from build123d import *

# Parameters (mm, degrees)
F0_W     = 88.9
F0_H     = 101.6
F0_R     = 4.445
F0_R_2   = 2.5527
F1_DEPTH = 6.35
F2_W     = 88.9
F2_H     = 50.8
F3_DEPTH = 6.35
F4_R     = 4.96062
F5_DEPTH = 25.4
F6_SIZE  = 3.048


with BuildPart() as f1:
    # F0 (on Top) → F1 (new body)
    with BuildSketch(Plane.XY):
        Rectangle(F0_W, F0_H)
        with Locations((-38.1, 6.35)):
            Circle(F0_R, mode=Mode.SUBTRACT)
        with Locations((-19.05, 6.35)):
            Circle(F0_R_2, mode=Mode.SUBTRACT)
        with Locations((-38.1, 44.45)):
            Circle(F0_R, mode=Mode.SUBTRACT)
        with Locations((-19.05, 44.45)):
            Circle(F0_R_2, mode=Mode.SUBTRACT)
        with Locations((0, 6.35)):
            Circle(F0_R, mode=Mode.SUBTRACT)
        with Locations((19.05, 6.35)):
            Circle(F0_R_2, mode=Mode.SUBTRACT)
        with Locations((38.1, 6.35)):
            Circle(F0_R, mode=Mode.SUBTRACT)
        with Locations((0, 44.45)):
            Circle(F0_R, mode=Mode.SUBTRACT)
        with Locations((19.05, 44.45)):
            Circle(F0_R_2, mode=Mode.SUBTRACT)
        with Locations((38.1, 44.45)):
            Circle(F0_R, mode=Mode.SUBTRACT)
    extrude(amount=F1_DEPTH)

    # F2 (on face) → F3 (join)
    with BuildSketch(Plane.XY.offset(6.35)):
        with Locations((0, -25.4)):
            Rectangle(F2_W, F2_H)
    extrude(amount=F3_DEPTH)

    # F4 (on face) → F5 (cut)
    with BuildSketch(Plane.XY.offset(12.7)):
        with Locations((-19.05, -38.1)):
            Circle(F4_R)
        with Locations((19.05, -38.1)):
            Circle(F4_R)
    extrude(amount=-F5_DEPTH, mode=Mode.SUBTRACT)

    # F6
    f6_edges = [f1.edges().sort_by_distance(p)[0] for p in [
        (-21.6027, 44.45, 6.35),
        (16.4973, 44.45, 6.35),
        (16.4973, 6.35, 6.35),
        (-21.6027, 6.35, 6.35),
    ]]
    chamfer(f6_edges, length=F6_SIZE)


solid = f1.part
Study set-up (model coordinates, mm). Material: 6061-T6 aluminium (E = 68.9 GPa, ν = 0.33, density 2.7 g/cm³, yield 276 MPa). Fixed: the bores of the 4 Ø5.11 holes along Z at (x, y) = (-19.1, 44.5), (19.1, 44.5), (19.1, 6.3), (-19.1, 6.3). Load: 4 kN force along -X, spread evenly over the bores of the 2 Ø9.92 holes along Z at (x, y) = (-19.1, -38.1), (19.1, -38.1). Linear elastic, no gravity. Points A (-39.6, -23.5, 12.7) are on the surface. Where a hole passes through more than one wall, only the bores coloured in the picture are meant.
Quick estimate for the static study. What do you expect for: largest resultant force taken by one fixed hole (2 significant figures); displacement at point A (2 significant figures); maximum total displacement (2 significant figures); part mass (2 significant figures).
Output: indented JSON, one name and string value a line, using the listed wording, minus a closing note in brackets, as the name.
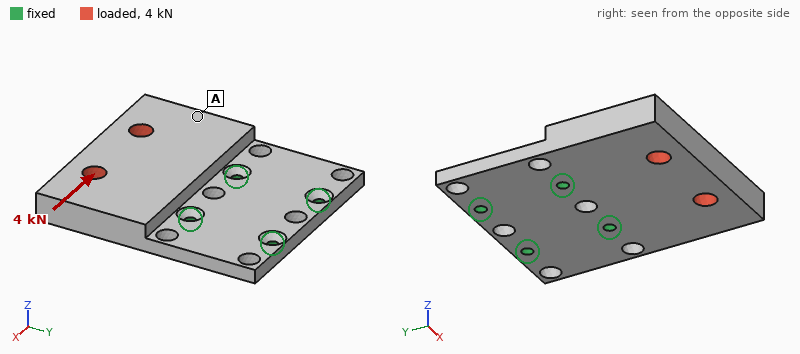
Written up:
{
  "largest resultant force taken by one fixed hole": "3.7 kN",
  "displacement at point A": "25 µm",
  "maximum total displacement": "40 µm",
  "part mass": "220 g"
}
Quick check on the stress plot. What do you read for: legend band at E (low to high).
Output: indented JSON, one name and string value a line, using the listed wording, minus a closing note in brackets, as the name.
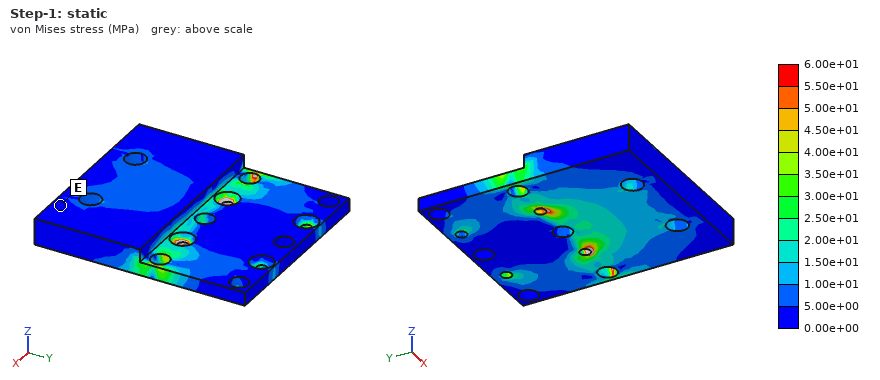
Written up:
{
  "legend band at E": "0.00e+00 to 5.00e+00 MPa"
}
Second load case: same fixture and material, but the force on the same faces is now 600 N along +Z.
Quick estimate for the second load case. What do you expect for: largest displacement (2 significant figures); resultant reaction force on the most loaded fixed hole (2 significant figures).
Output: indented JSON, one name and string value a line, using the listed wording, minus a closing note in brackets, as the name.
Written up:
{
  "largest displacement": "0.20 mm",
  "resultant reaction force on the most loaded fixed hole": "690 N"
}
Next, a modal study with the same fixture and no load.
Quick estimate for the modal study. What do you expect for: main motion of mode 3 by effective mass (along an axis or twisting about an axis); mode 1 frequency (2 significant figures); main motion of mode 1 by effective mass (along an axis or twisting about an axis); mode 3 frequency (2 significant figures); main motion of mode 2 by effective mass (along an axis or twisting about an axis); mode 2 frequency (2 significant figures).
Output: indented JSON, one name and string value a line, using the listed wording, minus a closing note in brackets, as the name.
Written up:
{
  "main motion of mode 3 by effective mass": "along X",
  "mode 1 frequency": "1100 Hz",
  "main motion of mode 1 by effective mass": "along Z",
  "mode 3 frequency": "5800 Hz",
  "main motion of mode 2 by effective mass": "twisting about Y",
  "mode 2 frequency": "2900 Hz"
}
